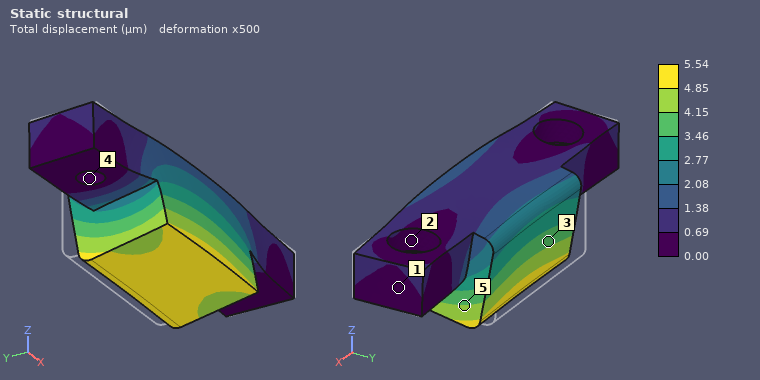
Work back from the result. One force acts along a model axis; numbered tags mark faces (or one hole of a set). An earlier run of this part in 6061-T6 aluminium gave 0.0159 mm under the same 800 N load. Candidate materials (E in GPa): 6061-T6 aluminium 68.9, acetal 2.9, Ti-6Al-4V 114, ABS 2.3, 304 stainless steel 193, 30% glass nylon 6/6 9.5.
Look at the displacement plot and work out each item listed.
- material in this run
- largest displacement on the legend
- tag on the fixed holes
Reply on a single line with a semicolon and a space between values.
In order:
304 stainless steel; 5.54 µm; 4
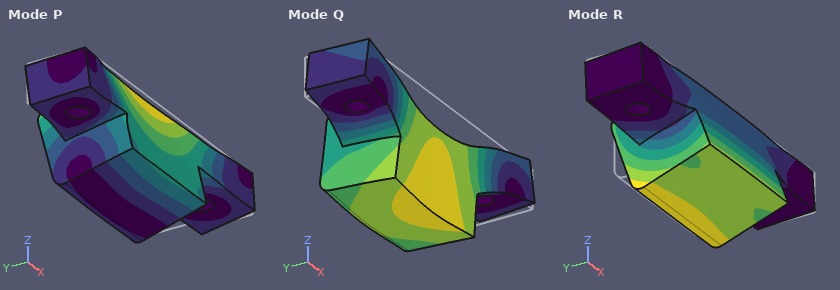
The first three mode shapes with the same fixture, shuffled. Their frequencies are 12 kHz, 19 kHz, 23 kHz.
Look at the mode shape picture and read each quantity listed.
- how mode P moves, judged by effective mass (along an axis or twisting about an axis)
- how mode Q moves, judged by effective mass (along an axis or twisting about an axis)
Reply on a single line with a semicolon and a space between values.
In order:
along Y; along Z
